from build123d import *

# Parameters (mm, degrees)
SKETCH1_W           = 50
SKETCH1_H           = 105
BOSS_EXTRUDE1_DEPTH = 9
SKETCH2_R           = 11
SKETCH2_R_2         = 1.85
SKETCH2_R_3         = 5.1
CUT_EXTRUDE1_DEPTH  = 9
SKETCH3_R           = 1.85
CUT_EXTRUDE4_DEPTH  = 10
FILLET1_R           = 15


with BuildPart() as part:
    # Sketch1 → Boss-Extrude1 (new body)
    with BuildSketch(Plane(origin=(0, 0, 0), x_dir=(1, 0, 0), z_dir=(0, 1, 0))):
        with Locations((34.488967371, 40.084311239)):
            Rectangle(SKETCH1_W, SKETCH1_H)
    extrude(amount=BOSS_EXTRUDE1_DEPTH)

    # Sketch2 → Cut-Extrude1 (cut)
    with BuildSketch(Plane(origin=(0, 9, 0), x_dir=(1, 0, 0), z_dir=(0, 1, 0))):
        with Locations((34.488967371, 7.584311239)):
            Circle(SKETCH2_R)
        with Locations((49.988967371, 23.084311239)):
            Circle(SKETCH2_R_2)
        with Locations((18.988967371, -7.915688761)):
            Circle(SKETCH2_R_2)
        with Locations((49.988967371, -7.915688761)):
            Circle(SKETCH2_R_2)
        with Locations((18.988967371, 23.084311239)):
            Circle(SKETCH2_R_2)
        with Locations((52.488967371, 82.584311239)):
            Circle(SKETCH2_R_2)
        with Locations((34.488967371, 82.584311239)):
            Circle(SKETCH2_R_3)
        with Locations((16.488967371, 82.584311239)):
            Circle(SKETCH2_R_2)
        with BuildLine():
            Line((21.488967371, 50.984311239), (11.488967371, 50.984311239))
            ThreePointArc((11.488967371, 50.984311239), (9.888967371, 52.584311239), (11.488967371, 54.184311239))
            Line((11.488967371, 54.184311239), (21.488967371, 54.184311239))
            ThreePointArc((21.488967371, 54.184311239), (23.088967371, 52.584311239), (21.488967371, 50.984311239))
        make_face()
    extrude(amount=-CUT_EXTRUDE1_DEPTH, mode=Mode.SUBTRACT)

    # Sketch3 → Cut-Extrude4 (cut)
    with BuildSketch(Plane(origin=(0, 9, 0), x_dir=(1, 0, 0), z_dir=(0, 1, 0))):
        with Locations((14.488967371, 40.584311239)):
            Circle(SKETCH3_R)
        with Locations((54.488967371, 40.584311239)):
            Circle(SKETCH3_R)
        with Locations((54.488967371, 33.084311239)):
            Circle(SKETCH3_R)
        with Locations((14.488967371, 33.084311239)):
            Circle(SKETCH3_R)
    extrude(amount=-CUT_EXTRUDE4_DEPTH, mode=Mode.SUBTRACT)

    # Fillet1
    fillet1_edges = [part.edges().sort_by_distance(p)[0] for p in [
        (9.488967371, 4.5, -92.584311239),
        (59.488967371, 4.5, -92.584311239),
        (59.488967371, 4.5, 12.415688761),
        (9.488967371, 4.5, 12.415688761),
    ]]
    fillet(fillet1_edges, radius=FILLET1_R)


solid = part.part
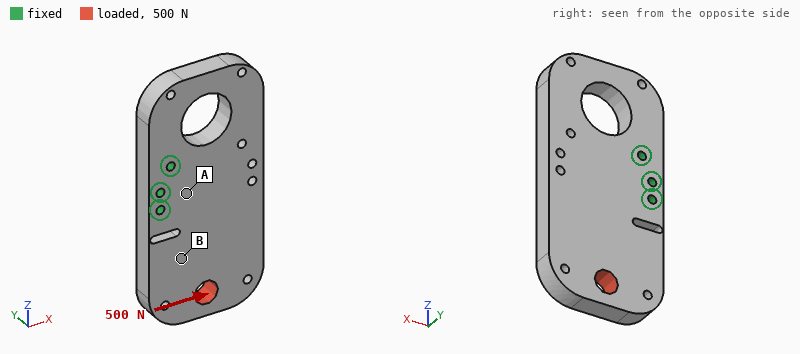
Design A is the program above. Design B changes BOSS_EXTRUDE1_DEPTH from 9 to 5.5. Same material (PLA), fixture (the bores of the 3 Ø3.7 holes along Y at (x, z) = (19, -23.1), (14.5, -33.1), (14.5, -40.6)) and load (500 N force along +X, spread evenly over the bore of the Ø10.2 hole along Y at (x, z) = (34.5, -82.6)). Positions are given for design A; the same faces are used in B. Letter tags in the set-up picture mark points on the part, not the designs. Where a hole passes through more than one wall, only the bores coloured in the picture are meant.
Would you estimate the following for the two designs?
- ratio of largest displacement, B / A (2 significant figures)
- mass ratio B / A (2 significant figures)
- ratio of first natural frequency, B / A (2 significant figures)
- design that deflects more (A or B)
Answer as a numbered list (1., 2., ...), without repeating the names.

1. 1.7
2. 0.61
3. 0.64
4. B
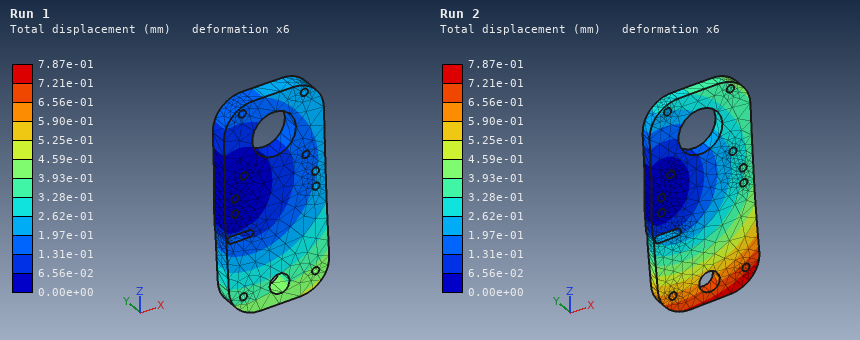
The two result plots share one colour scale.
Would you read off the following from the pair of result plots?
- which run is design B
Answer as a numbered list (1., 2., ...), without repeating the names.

1. Run 2
